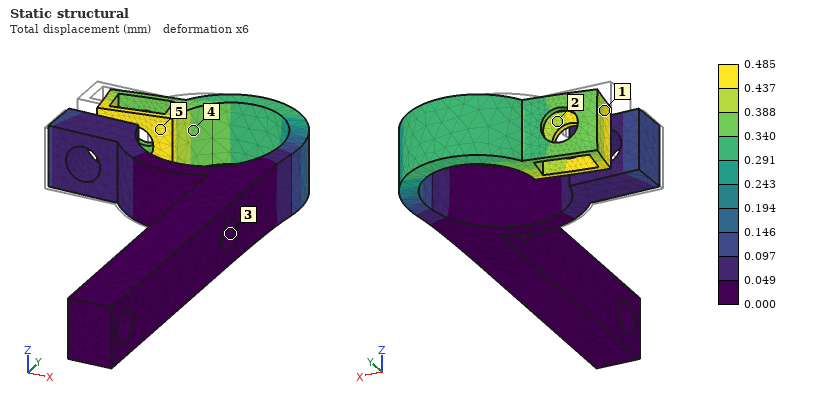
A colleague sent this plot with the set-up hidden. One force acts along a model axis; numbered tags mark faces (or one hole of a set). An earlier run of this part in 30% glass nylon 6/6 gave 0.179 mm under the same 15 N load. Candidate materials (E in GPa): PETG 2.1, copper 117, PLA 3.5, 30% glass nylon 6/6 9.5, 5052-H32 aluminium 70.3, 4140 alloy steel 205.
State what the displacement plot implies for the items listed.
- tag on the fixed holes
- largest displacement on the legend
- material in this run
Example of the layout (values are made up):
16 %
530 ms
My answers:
3
0.485 mm
PLA
